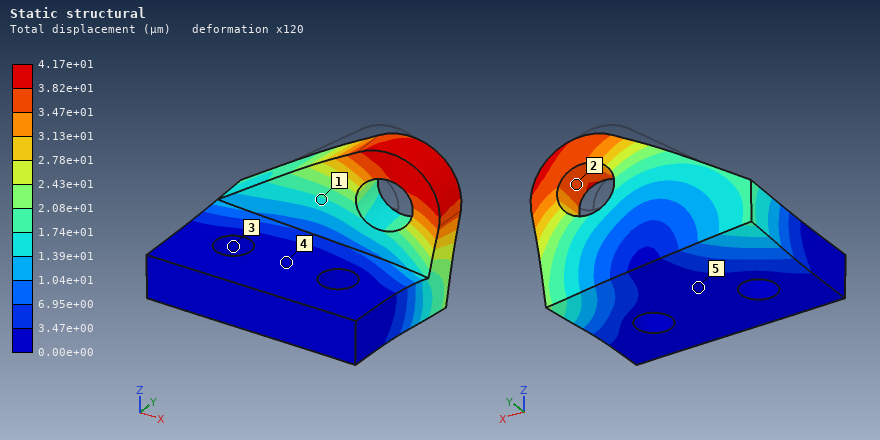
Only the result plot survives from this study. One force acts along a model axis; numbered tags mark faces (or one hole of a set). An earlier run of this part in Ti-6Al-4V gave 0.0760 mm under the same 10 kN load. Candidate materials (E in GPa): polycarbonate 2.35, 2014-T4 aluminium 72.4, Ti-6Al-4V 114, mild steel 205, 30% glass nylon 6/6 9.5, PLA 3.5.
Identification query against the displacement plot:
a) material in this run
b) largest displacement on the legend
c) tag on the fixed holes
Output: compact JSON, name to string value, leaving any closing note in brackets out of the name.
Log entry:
{"material in this run": "mild steel", "largest displacement on the legend": "4.17e+01 µm", "tag on the fixed holes": "3"}
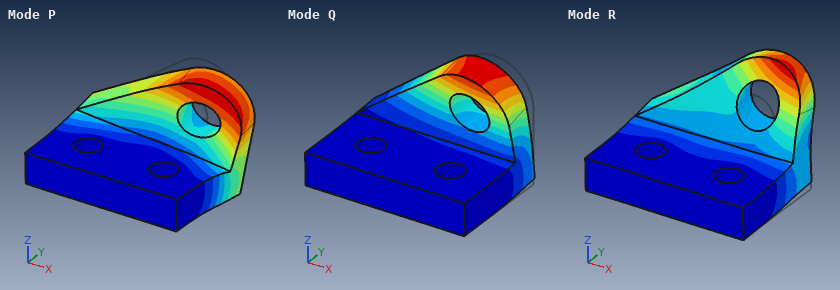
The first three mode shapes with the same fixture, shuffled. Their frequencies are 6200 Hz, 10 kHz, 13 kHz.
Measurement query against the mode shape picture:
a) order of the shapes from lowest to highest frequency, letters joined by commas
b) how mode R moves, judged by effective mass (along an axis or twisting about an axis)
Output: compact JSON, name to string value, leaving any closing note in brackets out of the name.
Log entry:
{"order of the shapes from lowest to highest frequency, letters joined by commas": "Q, P, R", "how mode R moves, judged by effective mass": "along Z"}
